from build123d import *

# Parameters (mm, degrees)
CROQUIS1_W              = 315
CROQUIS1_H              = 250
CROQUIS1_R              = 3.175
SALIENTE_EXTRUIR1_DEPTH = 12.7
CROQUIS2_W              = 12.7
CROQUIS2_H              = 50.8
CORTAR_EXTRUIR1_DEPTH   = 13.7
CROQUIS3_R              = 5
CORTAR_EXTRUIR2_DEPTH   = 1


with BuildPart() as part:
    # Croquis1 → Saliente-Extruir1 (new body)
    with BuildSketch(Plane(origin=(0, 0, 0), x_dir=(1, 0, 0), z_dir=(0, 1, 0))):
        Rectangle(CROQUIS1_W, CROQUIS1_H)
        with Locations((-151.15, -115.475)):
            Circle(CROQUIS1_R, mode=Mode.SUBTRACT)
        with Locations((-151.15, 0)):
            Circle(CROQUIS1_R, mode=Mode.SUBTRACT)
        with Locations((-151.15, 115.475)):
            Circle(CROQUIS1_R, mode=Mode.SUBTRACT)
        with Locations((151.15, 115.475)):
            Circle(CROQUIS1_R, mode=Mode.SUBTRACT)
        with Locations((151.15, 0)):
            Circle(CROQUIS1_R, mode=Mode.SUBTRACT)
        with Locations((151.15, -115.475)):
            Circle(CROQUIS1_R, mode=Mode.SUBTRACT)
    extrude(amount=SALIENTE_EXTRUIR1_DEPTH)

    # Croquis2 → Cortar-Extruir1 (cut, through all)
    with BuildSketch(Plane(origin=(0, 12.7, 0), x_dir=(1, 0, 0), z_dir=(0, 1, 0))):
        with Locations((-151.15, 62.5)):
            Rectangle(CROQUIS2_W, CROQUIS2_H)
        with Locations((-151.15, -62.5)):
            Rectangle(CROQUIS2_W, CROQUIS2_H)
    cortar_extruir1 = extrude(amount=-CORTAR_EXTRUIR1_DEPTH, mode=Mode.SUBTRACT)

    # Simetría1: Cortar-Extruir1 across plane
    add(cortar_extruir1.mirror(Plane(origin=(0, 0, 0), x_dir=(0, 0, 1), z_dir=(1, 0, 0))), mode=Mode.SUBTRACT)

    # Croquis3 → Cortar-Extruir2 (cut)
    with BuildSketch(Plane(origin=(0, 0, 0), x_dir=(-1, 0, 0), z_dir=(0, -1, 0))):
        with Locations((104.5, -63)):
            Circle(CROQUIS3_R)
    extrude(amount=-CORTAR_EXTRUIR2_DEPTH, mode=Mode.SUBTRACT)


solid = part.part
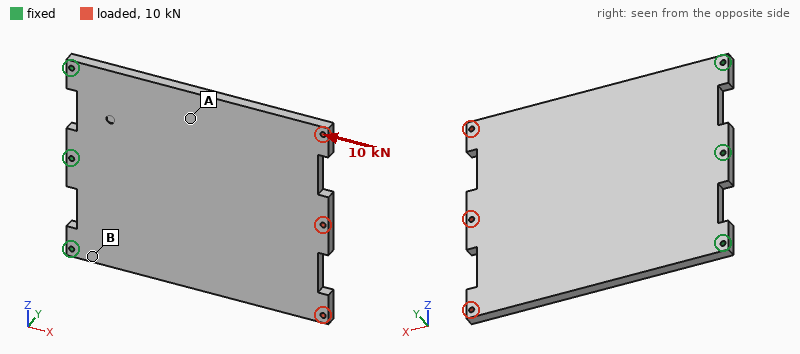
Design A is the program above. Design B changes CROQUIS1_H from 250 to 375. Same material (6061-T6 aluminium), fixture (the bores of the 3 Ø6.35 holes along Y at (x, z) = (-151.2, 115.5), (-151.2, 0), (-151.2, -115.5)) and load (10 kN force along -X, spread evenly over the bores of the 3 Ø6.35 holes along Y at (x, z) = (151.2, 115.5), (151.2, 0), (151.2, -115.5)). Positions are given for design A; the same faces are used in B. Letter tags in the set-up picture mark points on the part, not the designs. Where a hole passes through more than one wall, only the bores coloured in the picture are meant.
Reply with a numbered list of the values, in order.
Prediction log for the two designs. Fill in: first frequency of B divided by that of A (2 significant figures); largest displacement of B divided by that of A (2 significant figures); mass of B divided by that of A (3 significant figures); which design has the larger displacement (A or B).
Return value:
1. 0.95
2. 0.64
3. 1.52
4. A
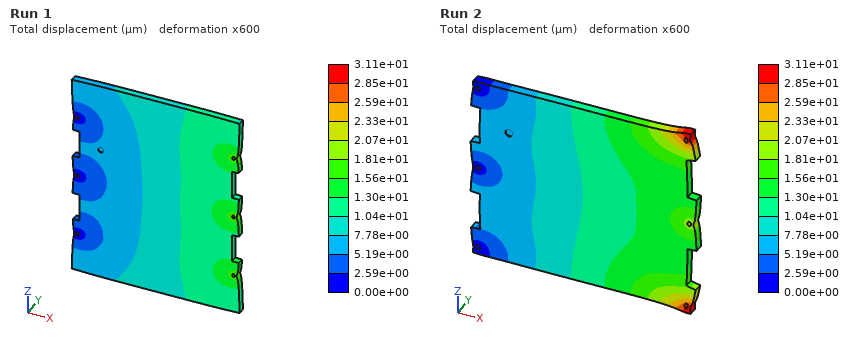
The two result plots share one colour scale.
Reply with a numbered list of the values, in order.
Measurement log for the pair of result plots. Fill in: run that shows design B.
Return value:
1. Run 1
